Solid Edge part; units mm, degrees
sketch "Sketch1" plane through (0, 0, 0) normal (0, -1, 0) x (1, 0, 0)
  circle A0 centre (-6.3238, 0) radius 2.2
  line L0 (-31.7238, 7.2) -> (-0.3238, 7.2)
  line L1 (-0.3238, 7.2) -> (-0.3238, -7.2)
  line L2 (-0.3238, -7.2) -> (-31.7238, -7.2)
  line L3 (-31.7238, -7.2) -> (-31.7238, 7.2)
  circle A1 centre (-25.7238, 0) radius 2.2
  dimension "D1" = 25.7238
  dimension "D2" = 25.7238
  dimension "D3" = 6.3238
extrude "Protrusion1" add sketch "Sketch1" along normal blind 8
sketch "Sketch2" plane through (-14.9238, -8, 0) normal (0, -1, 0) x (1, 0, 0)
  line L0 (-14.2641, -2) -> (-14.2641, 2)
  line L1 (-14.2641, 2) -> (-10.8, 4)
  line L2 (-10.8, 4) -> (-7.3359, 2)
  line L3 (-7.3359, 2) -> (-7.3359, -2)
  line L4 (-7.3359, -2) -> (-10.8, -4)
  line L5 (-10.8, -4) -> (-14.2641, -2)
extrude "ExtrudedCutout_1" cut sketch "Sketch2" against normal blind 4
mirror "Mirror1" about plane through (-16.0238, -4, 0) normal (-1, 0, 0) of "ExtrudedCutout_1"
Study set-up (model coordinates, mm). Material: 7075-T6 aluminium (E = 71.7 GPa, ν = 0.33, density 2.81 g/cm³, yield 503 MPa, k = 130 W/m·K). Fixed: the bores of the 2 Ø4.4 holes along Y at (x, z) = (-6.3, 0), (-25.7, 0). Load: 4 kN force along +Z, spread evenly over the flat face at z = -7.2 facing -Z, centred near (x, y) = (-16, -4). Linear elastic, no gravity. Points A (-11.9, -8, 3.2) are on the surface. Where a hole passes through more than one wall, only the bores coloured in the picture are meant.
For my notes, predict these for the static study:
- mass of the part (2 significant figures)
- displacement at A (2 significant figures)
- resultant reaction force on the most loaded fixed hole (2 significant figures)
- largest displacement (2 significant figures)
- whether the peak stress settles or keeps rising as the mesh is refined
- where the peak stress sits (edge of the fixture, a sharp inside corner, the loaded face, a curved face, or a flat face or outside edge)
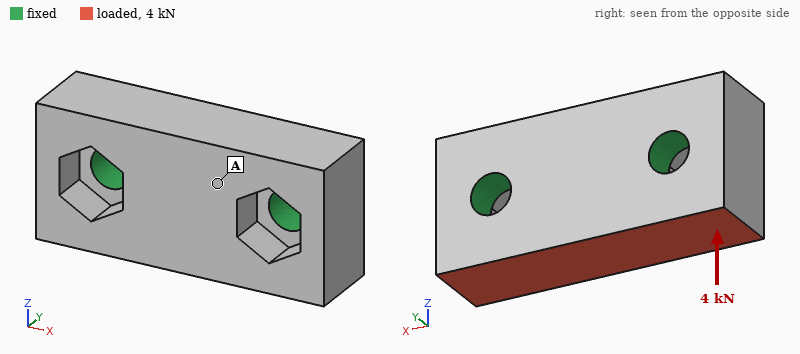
8.9 g
8.5 µm
2.0 kN
13 µm
keeps rising
edge of the fixture
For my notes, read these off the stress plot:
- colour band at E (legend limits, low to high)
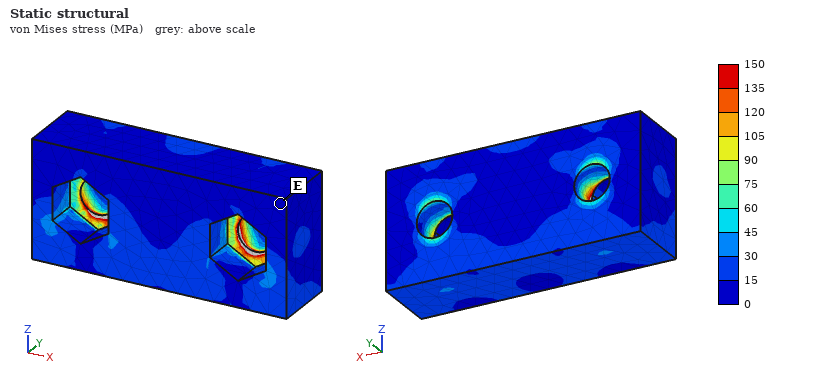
0 to 15 MPa
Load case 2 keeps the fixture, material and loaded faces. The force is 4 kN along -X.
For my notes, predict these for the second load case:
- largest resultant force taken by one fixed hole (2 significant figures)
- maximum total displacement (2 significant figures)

2.3 kN
13 µm
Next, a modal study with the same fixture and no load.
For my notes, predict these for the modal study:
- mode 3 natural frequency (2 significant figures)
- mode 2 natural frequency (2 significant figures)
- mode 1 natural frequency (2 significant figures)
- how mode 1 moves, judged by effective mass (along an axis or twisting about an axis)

48 kHz
47 kHz
31 kHz
along Z
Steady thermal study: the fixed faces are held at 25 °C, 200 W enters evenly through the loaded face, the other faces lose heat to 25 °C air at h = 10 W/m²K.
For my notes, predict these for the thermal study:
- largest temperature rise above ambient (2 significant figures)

71 K
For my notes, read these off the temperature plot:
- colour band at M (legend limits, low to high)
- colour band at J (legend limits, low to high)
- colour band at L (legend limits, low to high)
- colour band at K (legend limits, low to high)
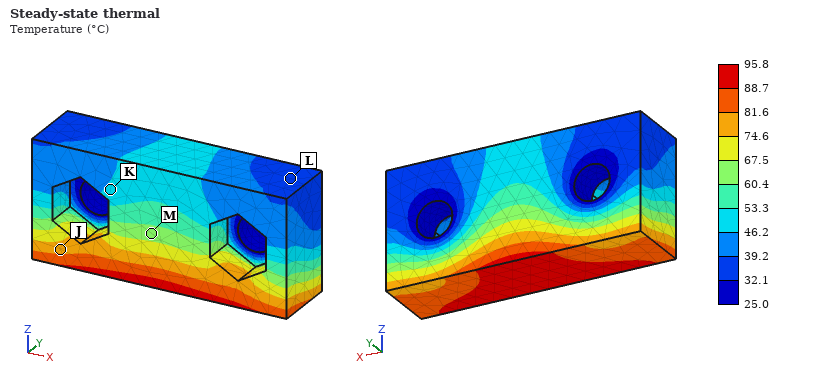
60.4 to 67.5 °C
74.6 to 81.6 °C
32.1 to 39.2 °C
46.2 to 53.3 °C
